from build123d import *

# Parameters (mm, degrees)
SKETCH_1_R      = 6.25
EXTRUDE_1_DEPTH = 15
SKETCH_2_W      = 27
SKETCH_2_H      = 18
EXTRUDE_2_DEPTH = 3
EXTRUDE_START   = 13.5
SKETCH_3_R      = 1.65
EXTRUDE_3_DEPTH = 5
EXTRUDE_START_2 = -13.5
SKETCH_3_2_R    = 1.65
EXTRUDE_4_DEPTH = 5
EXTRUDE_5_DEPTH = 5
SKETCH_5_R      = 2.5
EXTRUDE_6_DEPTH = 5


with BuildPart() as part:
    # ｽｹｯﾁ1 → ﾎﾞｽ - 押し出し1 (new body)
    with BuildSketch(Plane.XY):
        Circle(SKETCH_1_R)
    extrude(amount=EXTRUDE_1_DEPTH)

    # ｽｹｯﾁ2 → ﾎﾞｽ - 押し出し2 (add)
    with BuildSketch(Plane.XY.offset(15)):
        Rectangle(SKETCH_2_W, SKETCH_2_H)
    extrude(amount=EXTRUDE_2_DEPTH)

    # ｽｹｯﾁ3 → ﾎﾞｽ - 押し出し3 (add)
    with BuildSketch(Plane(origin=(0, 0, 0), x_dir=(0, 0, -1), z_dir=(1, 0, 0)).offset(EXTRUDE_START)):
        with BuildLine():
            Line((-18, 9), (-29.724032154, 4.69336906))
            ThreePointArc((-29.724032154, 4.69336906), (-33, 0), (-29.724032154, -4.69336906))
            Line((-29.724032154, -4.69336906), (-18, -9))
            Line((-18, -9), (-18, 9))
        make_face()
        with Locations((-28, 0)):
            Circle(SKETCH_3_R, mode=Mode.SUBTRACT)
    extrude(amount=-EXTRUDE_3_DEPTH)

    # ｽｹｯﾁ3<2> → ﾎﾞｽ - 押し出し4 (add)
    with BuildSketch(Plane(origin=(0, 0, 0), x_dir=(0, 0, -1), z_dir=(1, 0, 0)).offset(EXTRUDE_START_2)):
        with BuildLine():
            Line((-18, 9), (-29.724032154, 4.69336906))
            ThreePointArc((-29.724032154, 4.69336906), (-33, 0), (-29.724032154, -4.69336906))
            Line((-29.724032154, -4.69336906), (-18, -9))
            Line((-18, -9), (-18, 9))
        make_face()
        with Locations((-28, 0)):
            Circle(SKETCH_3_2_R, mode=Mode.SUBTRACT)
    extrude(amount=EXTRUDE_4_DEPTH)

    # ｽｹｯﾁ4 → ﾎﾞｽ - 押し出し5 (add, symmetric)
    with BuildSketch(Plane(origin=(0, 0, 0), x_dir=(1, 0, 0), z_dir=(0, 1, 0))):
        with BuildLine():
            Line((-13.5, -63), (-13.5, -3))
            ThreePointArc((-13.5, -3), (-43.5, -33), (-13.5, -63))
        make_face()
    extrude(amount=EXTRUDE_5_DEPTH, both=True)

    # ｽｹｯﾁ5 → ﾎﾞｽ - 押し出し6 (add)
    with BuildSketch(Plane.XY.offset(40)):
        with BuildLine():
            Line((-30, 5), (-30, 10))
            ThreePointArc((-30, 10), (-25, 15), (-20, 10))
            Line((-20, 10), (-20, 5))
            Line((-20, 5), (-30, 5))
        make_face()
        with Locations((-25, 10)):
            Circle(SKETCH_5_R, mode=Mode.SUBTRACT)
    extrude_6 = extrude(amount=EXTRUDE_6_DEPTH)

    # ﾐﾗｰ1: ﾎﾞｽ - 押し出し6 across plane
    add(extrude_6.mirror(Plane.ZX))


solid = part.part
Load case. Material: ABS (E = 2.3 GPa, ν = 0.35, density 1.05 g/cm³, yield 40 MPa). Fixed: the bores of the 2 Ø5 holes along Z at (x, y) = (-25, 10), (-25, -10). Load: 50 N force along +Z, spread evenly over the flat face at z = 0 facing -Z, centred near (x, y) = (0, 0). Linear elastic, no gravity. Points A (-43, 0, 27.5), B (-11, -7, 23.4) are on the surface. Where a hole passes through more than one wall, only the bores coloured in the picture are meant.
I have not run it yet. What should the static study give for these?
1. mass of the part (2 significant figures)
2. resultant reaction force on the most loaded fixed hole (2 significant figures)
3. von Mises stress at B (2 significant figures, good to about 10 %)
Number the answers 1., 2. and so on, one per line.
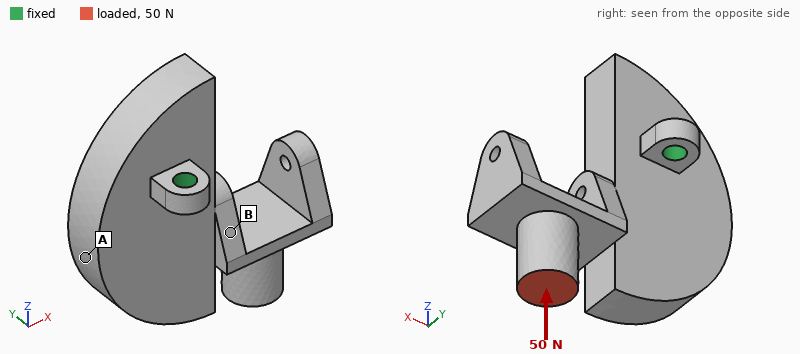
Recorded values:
1. 21 g
2. 25 N
3. 2.3 MPa
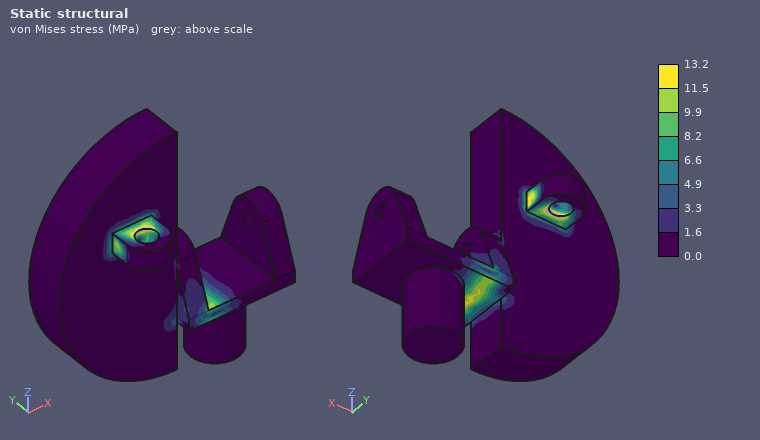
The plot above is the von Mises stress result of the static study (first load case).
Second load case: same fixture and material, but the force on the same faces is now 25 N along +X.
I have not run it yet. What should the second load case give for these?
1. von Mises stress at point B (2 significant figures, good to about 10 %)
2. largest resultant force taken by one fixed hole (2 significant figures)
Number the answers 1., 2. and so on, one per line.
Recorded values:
1. 1.7 MPa
2. 13 N
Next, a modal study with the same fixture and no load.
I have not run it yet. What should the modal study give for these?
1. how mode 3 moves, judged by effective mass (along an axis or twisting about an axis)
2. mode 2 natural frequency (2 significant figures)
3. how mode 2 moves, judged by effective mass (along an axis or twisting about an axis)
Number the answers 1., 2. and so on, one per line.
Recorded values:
1. along X
2. 780 Hz
3. along Y
